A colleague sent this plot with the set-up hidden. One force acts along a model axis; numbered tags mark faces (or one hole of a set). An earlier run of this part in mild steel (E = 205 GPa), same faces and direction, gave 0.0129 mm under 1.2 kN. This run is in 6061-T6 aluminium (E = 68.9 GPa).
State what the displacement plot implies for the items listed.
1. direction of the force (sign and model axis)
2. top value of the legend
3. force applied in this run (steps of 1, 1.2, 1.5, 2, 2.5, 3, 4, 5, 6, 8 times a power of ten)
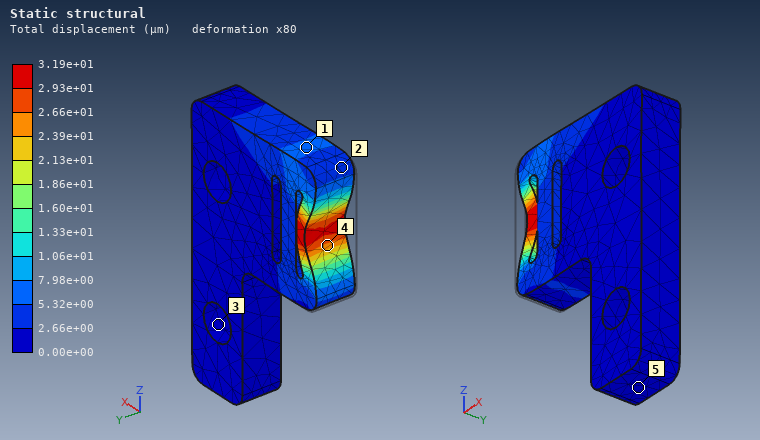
+X
3.19e+01 µm
1 kN
